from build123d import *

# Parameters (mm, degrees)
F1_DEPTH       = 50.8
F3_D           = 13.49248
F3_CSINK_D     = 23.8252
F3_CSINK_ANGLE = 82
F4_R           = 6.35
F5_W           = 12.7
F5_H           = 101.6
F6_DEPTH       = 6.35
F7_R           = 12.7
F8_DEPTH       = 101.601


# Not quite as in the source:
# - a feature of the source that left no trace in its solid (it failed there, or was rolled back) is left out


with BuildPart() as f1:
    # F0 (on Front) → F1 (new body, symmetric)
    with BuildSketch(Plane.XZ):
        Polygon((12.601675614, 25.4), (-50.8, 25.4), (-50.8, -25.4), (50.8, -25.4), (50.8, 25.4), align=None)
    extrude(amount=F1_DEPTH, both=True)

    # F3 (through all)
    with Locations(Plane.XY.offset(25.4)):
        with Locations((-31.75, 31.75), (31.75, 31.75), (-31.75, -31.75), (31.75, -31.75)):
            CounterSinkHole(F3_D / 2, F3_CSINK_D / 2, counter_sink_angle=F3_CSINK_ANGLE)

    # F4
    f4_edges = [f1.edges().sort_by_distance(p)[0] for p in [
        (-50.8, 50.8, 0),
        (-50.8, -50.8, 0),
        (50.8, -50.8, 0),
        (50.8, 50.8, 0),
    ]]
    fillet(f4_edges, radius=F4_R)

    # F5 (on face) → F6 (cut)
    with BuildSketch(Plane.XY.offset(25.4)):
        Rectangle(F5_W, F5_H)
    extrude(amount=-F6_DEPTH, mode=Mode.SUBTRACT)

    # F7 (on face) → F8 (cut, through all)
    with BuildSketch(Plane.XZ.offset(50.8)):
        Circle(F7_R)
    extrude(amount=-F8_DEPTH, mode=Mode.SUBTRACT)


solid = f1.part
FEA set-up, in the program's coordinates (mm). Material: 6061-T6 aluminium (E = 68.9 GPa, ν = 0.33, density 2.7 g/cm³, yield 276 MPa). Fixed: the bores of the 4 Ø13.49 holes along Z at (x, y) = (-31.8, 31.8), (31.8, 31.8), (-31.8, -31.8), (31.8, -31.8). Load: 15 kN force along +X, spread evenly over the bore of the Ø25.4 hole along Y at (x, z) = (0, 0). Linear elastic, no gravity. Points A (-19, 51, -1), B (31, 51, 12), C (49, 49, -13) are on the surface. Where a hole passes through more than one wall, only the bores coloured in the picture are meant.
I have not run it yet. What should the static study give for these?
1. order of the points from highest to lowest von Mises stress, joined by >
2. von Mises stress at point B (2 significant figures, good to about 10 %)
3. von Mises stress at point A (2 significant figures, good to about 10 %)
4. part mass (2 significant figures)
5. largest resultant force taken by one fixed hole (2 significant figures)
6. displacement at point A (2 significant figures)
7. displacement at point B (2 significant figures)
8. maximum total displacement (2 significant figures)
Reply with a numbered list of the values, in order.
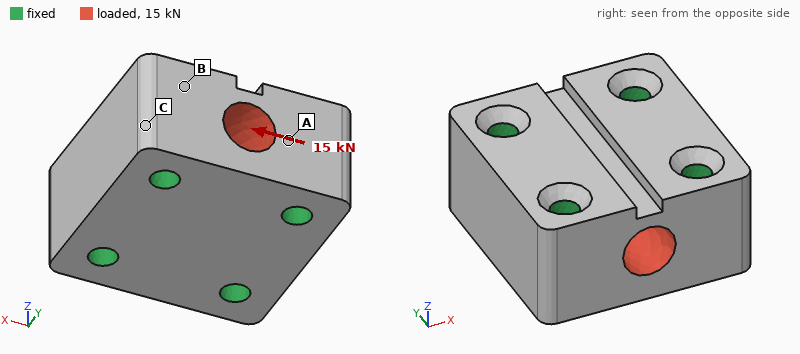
1. A > B > C
2. 0.91 MPa
3. 1.7 MPa
4. 1.2 kg
5. 3.8 kN
6. 0.54 µm
7. 0.29 µm
8. 1.2 µm
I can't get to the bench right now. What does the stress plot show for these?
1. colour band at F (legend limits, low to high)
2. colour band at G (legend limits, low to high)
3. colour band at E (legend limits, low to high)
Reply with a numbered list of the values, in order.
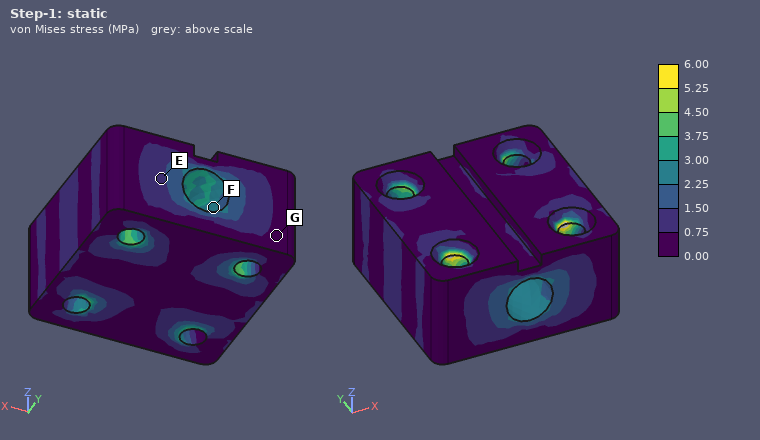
1. 2.25 to 3.00 MPa
2. 0.00 to 0.75 MPa
3. 0.75 to 1.50 MPa
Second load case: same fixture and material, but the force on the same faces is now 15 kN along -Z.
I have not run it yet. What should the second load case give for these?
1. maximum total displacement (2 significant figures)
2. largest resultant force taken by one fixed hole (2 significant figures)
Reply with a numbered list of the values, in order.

1. 3.5 µm
2. 3.8 kN
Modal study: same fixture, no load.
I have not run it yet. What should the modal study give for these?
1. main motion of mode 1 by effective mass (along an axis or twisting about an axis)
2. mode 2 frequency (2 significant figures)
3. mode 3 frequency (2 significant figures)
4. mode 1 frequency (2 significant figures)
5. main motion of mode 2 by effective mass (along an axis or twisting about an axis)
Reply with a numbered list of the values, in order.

1. along Z
2. 22 kHz
3. 23 kHz
4. 20 kHz
5. along X
